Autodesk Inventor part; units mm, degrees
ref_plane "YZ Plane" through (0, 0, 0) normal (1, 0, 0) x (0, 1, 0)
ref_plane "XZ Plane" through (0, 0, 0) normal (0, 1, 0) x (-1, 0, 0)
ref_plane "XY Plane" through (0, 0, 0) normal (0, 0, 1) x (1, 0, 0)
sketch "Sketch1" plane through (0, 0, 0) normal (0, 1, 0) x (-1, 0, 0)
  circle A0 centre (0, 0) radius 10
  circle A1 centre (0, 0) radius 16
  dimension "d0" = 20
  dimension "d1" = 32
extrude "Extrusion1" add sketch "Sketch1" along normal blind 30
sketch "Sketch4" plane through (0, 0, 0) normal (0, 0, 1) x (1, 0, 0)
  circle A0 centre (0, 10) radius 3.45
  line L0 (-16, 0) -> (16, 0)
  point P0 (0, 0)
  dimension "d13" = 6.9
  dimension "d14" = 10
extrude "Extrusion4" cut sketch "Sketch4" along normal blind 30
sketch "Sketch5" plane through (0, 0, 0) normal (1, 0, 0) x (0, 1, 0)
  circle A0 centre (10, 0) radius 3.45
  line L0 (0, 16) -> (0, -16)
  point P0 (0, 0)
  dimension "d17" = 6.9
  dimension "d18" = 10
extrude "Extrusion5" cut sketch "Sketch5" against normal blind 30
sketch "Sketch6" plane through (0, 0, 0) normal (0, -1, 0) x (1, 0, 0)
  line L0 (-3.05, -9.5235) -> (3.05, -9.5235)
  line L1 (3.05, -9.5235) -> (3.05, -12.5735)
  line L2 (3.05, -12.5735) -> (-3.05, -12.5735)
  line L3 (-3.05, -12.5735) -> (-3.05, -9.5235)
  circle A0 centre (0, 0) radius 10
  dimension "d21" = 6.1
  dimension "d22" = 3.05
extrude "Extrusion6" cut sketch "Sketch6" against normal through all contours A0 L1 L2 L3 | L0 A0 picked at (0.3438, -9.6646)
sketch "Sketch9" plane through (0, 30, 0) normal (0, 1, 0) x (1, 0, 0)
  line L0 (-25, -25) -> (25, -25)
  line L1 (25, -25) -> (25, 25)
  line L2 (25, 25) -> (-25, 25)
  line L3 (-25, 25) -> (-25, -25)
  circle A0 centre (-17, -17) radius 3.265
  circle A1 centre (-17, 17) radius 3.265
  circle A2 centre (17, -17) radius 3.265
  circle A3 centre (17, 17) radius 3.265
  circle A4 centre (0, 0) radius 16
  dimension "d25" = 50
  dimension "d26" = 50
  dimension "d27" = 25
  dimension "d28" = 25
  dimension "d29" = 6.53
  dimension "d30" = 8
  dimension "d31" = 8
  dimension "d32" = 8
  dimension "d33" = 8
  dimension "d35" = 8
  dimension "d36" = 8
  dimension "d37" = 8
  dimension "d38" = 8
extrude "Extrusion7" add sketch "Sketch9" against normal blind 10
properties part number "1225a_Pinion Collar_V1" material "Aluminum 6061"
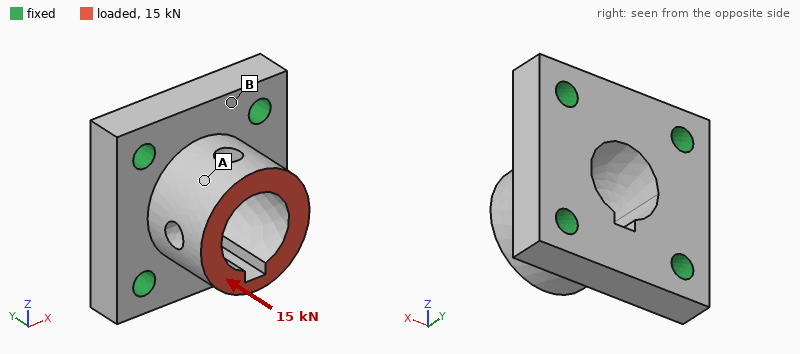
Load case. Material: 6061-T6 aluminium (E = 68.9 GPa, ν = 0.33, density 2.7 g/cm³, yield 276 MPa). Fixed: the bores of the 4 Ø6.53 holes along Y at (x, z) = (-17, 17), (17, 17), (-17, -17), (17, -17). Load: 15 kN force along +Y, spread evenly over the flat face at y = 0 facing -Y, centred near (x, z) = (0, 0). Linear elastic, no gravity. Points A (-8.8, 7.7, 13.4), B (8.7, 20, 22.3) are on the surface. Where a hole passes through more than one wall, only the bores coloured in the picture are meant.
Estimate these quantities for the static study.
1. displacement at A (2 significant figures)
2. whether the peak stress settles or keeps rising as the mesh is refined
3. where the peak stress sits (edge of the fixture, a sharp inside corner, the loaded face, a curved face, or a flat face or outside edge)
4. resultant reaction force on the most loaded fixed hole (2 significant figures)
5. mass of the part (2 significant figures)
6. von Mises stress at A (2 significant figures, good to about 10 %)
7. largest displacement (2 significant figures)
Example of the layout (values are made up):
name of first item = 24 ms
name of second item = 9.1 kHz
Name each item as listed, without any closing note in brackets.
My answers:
displacement at A = 20 µm
whether the peak stress settles or keeps rising as the mesh is refined = keeps rising
where the peak stress sits = edge of the fixture
resultant reaction force on the most loaded fixed hole = 4.0 kN
mass of the part = 79 g
von Mises stress at A = 29 MPa
largest displacement = 27 µm
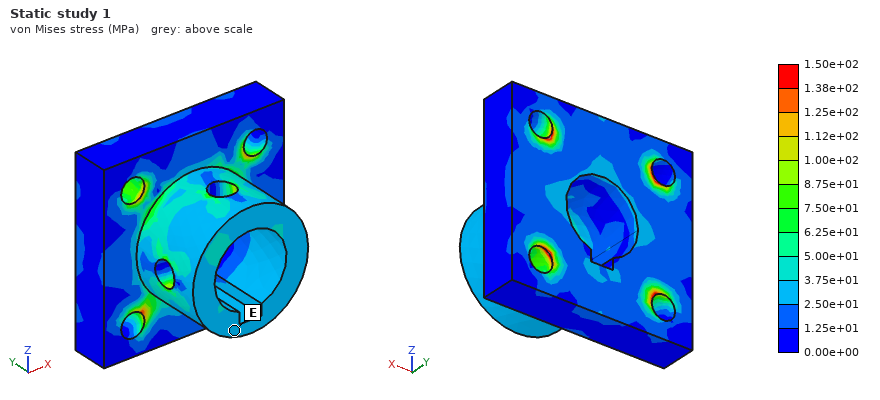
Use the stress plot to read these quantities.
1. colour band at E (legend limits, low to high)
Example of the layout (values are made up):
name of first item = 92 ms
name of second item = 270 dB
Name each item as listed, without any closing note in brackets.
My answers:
colour band at E = 2.50e+01 to 3.75e+01 MPa
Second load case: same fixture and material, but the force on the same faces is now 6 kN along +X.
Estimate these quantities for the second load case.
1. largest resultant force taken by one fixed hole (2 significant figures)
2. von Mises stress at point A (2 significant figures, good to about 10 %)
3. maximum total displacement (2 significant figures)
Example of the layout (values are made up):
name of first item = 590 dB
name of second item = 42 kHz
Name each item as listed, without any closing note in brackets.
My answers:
largest resultant force taken by one fixed hole = 2.9 kN
von Mises stress at point A = 36 MPa
maximum total displacement = 60 µm
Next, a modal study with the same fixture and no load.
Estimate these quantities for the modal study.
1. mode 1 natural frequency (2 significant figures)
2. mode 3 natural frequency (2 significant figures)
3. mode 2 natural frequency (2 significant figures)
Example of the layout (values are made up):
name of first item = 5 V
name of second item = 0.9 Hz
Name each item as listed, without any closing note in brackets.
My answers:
mode 1 natural frequency = 18 kHz
mode 3 natural frequency = 23 kHz
mode 2 natural frequency = 18 kHz
